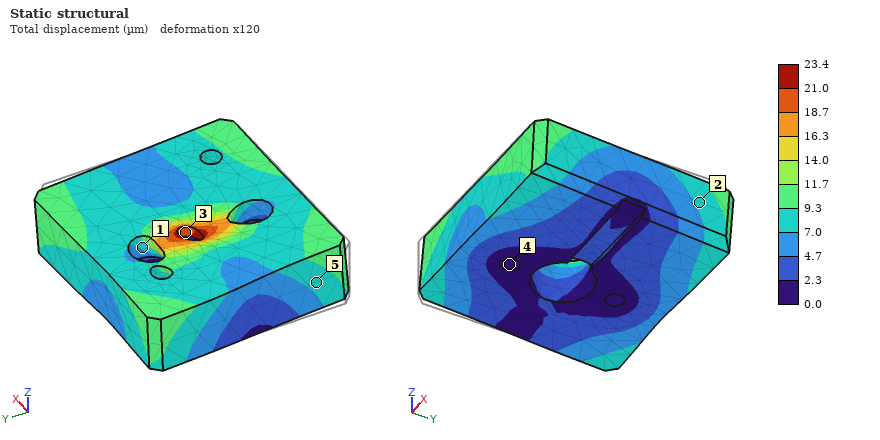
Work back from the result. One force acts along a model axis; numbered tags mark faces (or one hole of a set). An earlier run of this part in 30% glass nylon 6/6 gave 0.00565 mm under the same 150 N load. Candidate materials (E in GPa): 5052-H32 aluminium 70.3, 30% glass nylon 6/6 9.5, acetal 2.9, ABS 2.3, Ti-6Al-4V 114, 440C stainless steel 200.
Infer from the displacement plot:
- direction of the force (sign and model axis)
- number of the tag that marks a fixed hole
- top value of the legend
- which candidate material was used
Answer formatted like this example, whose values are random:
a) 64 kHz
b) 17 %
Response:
a) +Y
b) 4
c) 23.4 µm
d) ABS
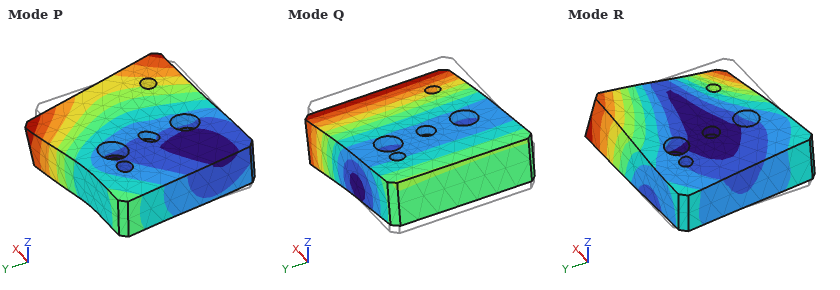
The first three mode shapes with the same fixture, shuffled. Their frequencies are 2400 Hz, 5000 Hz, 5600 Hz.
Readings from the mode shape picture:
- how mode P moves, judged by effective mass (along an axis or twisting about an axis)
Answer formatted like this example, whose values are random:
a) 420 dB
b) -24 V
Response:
a) along Y
